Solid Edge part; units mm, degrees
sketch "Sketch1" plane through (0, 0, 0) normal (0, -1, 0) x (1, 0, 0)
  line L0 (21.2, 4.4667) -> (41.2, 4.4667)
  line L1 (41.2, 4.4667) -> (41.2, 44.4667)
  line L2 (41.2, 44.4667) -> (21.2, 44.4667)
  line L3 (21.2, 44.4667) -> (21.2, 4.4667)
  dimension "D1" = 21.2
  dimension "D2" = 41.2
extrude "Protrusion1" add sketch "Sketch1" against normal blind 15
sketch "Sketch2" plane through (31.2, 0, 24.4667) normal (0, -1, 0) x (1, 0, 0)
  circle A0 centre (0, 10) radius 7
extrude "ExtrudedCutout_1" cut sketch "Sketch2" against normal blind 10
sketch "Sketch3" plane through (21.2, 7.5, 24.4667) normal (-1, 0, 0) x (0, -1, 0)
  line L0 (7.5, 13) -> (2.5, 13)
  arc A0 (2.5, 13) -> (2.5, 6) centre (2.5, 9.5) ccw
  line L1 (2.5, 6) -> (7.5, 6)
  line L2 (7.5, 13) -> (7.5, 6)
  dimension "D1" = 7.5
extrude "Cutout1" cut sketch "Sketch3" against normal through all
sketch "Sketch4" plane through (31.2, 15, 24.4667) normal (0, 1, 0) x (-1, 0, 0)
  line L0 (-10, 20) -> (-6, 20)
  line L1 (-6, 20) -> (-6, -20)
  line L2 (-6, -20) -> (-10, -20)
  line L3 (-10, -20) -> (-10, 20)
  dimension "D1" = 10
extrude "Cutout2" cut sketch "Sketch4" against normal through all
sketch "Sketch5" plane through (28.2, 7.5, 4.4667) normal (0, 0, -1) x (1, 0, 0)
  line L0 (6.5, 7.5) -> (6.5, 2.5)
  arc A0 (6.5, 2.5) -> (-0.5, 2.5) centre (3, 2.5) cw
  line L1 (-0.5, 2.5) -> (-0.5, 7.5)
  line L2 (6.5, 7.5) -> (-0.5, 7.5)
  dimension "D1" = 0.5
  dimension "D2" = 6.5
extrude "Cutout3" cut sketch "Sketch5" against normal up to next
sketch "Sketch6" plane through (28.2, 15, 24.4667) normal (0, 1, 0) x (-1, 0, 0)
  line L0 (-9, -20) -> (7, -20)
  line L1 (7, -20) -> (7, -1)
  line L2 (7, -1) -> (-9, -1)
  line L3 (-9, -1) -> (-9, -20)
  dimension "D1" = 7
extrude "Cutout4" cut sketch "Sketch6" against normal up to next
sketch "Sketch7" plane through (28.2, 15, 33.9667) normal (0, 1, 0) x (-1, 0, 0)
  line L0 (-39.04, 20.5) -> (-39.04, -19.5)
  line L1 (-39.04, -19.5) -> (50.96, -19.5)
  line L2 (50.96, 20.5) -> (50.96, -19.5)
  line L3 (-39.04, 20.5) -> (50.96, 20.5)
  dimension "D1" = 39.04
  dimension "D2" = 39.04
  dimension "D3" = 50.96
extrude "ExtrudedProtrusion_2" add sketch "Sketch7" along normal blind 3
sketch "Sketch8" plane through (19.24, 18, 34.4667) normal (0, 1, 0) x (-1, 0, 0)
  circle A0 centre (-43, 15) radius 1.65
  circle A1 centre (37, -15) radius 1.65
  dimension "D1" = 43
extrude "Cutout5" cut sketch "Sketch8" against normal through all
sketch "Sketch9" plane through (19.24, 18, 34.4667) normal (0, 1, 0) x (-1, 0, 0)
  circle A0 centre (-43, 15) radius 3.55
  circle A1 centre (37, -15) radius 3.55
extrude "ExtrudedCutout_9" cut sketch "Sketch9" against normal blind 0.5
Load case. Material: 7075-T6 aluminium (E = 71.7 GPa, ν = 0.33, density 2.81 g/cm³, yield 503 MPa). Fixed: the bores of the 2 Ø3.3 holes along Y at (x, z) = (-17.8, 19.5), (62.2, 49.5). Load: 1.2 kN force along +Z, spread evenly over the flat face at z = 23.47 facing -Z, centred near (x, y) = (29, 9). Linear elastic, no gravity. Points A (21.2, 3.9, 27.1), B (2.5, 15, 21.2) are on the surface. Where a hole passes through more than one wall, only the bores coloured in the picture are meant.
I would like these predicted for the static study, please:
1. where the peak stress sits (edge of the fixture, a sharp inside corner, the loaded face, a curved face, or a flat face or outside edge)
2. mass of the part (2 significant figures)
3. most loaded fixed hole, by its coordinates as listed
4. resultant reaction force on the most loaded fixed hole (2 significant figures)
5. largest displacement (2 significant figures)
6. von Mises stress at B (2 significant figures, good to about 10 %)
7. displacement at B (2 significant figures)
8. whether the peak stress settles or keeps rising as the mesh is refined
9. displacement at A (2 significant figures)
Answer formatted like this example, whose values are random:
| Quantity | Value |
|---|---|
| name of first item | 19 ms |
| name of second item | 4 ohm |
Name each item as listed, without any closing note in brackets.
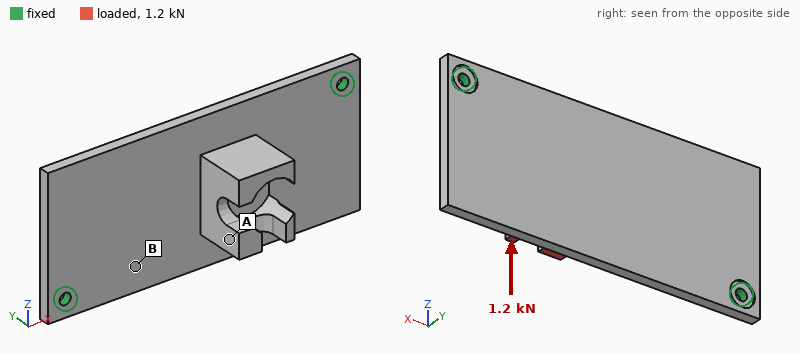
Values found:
| Quantity | Value |
|---|---|
| where the peak stress sits | edge of the fixture |
| mass of the part | 39 g |
| most loaded fixed hole, by its coordinates as listed | (62.2, 49.5) |
| resultant reaction force on the most loaded fixed hole | 710 N |
| largest displacement | 0.61 mm |
| von Mises stress at B | 86 MPa |
| displacement at B | 0.13 mm |
| whether the peak stress settles or keeps rising as the mesh is refined | keeps rising |
| displacement at A | 0.39 mm |
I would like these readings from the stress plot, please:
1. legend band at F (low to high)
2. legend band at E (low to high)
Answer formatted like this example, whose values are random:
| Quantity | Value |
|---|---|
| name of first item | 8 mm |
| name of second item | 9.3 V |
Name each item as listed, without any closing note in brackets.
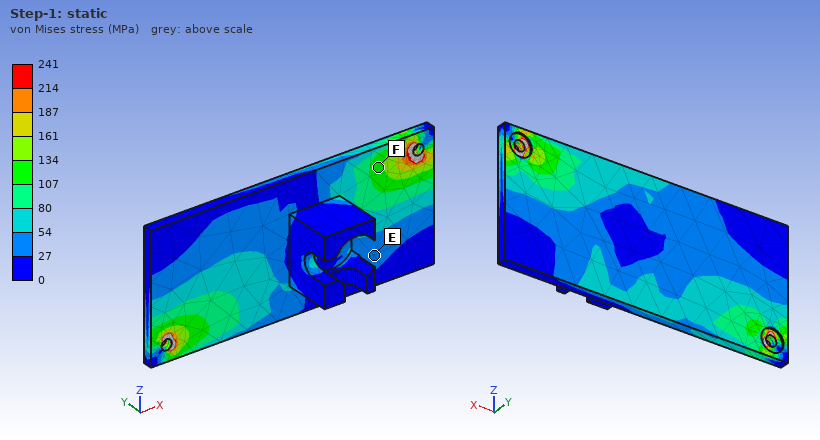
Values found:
| Quantity | Value |
|---|---|
| legend band at F | 107 to 134 MPa |
| legend band at E | 27 to 54 MPa |
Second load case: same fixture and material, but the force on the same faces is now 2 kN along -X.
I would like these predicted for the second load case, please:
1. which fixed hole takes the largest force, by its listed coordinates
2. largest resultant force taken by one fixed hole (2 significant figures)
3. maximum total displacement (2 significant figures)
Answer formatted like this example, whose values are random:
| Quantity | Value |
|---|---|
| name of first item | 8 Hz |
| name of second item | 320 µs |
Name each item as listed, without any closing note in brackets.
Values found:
| Quantity | Value |
|---|---|
| which fixed hole takes the largest force, by its listed coordinates | (62.2, 49.5) |
| largest resultant force taken by one fixed hole | 1.1 kN |
| maximum total displacement | 0.43 mm |
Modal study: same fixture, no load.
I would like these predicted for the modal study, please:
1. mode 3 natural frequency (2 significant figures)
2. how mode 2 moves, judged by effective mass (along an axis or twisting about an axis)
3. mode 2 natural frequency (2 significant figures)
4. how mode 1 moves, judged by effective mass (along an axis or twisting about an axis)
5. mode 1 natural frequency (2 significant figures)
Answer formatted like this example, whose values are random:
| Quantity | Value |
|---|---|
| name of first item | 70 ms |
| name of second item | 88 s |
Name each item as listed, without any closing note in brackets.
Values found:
| Quantity | Value |
|---|---|
| mode 3 natural frequency | 3300 Hz |
| how mode 2 moves, judged by effective mass | along Y |
| mode 2 natural frequency | 1400 Hz |
| how mode 1 moves, judged by effective mass | along Y |
| mode 1 natural frequency | 1300 Hz |
